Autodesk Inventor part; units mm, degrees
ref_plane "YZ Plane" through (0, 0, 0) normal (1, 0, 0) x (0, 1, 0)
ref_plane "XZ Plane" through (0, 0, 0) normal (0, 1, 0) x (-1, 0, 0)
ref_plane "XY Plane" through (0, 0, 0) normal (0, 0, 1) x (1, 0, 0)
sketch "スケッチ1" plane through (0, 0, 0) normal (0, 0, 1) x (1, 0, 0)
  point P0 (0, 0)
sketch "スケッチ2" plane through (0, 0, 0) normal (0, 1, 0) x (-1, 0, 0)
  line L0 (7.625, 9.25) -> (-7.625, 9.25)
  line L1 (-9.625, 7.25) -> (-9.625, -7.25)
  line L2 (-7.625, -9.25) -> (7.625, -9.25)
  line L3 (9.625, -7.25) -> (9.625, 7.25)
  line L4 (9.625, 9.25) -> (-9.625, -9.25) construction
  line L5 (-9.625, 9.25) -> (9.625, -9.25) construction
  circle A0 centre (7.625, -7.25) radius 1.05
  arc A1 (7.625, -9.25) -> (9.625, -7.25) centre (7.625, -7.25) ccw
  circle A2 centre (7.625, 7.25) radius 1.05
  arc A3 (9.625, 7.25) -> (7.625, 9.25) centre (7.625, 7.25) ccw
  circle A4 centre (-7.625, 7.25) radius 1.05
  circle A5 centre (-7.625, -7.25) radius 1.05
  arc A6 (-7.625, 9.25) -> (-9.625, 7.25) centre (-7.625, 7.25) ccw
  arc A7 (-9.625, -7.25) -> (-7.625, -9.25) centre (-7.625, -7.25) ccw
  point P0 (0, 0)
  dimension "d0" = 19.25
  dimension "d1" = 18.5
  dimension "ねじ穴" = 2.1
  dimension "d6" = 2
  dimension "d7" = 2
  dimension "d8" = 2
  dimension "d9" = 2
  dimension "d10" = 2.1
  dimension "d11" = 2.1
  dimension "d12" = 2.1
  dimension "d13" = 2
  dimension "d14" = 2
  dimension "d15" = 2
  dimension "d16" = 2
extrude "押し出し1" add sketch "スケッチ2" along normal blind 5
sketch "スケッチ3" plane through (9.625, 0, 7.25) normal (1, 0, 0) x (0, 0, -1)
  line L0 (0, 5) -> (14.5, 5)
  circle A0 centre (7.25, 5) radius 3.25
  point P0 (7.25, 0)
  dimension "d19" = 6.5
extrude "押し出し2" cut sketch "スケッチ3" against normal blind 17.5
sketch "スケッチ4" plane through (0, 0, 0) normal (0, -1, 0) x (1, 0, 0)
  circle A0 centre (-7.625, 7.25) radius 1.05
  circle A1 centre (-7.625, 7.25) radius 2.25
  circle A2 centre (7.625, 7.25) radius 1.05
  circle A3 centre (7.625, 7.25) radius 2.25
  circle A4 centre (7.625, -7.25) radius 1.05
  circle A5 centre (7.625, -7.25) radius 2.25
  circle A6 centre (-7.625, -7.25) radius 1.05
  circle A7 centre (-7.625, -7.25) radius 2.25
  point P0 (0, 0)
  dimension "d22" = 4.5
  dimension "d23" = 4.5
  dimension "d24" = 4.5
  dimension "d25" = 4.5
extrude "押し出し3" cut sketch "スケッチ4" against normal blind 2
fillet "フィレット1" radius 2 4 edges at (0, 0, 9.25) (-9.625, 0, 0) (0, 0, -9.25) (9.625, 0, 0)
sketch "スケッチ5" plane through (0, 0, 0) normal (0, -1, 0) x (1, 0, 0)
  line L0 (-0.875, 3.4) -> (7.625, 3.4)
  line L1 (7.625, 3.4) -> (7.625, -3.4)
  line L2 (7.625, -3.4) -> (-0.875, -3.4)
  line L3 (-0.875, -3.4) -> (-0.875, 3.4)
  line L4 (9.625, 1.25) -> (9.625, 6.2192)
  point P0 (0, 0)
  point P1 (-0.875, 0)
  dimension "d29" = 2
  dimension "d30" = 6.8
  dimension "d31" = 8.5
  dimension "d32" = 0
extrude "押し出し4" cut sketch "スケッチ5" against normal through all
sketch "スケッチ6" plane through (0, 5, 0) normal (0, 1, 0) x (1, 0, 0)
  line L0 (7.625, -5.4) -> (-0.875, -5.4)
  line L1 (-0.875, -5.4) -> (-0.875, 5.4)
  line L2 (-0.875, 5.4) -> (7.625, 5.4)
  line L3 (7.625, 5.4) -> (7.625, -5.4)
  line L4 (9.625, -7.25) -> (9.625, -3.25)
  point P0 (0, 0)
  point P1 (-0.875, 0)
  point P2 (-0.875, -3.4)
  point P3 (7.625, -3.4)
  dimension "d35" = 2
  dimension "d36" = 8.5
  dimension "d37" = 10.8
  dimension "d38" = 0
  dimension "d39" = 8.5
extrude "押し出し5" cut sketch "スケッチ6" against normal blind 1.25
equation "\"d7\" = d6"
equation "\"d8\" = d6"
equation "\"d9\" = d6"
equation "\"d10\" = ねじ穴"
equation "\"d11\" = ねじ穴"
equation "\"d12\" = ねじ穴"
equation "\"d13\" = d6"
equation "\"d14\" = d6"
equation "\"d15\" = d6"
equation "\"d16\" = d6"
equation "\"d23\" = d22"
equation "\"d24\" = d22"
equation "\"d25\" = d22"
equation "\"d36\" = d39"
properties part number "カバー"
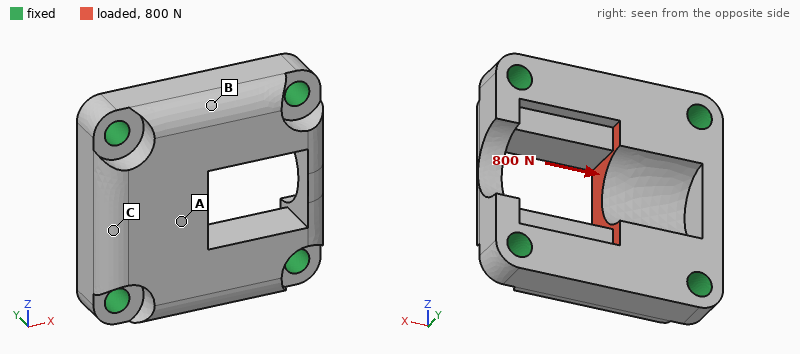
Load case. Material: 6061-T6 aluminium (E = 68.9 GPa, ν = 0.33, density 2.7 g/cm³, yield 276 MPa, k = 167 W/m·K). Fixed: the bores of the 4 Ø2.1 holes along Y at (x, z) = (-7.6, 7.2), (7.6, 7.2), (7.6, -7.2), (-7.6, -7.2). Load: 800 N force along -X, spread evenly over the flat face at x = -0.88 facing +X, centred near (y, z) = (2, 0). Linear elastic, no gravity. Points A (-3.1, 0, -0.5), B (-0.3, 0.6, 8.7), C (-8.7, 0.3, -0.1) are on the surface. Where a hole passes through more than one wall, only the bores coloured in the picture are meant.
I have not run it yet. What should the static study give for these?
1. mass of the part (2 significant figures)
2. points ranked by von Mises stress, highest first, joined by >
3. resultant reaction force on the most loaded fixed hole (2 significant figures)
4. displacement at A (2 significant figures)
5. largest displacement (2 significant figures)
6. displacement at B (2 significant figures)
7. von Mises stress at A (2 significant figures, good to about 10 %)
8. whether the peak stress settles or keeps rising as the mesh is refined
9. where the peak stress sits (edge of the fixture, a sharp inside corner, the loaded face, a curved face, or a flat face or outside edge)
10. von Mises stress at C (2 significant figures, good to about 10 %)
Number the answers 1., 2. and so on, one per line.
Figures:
1. 2.9 g
2. A > C > B
3. 250 N
4. 4.6 µm
5. 6.0 µm
6. 0.90 µm
7. 29 MPa
8. keeps rising
9. edge of the fixture
10. 15 MPa
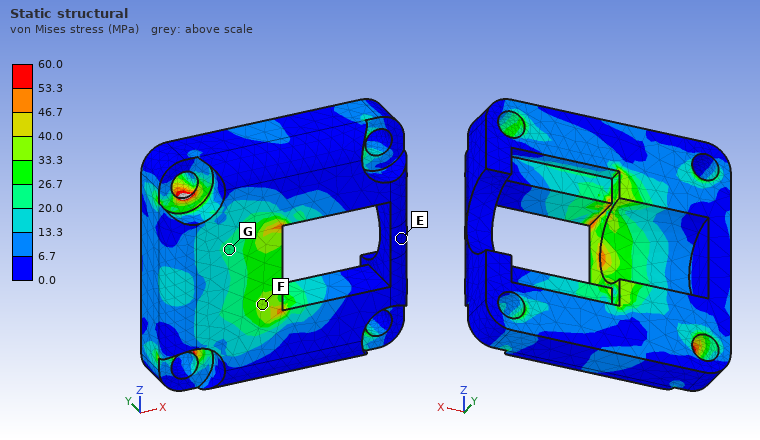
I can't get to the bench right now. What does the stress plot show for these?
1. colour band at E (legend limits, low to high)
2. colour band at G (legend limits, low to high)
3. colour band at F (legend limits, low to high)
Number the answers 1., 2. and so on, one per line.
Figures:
1. 0.0 to 6.7 MPa
2. 20.0 to 26.7 MPa
3. 33.3 to 40.0 MPa
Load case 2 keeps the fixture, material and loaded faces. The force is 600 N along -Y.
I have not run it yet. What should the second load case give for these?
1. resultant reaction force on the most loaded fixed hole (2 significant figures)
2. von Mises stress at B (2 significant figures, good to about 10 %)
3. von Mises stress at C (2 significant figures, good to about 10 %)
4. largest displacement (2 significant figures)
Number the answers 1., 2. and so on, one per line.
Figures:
1. 290 N
2. 16 MPa
3. 16 MPa
4. 18 µm
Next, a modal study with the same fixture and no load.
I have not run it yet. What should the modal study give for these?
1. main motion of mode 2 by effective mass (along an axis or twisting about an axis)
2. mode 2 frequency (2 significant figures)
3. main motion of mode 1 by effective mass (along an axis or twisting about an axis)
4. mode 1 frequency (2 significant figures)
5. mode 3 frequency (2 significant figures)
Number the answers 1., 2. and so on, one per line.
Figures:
1. along Z
2. 60 kHz
3. along Y
4. 54 kHz
5. 68 kHz
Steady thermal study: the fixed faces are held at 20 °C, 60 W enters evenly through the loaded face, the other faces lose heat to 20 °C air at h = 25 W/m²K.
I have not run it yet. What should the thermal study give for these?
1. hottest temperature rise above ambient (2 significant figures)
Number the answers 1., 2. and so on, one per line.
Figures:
1. 67 K
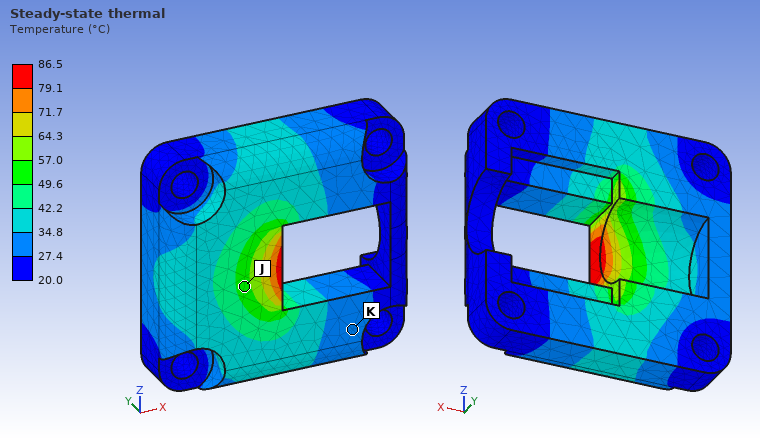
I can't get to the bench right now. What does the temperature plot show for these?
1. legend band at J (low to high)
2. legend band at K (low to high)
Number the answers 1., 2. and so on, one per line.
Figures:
1. 49.6 to 57.0 °C
2. 27.4 to 34.8 °C
